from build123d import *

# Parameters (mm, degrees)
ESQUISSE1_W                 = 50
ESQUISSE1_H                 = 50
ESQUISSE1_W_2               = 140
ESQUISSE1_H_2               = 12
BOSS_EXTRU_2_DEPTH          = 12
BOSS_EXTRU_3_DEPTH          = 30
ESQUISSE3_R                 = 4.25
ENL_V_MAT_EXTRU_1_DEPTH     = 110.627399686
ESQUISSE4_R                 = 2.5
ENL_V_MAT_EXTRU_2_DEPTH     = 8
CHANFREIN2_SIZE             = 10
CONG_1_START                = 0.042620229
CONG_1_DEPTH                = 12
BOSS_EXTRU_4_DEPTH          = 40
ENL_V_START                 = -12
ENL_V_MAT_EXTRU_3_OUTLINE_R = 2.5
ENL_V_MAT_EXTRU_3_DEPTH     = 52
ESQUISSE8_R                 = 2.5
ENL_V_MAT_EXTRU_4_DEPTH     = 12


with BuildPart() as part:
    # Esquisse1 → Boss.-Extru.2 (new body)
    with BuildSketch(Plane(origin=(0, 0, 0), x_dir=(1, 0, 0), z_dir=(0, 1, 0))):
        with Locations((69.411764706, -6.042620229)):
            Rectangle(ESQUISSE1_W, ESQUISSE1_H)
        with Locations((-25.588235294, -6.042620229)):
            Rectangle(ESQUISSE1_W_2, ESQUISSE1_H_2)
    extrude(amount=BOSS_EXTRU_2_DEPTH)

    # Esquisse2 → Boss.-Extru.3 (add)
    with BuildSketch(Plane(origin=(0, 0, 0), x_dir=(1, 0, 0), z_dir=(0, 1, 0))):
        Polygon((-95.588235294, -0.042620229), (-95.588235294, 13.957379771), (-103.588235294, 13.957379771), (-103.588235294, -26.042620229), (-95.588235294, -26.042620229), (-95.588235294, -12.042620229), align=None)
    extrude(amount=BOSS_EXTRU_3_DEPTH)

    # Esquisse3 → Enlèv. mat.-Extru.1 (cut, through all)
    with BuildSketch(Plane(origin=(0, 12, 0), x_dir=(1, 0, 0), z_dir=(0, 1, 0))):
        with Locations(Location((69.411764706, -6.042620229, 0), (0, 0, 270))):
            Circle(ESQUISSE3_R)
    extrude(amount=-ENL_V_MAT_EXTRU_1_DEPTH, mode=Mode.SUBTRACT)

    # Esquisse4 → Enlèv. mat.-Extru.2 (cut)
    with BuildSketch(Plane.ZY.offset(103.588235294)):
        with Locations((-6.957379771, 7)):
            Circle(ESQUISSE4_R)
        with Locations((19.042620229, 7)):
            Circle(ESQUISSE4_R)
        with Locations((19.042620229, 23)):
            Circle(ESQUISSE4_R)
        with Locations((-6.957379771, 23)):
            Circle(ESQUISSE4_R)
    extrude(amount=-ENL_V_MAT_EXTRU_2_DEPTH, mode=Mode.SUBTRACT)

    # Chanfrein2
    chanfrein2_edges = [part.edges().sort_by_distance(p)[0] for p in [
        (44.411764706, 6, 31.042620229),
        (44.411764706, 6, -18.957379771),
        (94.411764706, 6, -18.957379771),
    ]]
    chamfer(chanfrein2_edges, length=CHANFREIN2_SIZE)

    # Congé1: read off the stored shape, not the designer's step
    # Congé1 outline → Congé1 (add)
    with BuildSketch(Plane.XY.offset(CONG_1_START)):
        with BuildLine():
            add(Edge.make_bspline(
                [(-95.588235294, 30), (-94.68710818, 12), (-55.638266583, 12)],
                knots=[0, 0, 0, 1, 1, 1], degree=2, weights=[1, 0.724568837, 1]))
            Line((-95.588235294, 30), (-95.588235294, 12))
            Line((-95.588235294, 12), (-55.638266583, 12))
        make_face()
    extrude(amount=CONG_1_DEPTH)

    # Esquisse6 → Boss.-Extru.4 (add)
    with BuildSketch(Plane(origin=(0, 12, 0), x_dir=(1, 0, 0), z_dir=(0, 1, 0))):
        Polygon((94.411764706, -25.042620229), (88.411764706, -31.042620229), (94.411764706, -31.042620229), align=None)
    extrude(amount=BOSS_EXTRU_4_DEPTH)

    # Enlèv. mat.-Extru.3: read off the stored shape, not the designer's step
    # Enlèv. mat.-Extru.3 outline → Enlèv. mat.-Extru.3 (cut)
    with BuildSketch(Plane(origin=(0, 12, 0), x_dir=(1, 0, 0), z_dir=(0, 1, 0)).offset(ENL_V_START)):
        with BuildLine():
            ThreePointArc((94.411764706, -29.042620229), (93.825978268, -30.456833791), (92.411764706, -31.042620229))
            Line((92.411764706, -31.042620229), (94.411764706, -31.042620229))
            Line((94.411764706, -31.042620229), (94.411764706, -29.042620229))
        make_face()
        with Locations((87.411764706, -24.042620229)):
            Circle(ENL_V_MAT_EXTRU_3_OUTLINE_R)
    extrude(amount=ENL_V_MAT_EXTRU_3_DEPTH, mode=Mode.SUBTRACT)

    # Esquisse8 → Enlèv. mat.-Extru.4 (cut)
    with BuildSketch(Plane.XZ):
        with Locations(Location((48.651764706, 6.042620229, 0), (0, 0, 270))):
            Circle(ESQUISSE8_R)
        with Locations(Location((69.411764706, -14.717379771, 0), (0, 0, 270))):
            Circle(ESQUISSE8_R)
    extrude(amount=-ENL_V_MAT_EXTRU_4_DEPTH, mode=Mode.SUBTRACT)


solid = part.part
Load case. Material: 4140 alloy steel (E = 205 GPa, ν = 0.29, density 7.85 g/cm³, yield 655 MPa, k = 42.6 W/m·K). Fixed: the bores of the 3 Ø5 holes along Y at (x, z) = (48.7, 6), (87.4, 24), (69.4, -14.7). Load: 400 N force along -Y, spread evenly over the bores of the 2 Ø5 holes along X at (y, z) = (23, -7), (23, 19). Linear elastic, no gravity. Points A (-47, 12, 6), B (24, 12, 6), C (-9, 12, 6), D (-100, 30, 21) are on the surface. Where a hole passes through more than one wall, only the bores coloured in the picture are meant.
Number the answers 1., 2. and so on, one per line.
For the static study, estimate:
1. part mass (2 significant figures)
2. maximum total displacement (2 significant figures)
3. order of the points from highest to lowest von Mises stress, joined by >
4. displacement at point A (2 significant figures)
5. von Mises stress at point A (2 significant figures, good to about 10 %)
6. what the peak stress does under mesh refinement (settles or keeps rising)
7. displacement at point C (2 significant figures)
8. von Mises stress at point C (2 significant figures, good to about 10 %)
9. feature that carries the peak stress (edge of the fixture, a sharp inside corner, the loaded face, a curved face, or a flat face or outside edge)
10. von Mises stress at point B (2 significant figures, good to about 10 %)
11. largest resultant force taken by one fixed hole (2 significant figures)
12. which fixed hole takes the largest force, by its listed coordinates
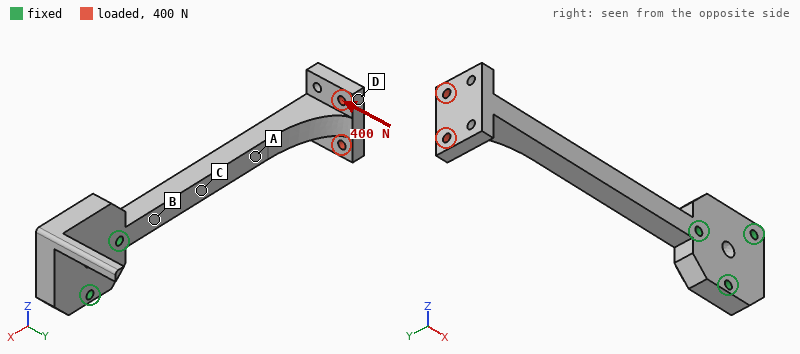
1. 460 g
2. 1.3 mm
3. B > C > A > D
4. 0.58 mm
5. 73 MPa
6. keeps rising
7. 0.23 mm
8. 130 MPa
9. edge of the fixture
10. 170 MPa
11. 840 N
12. (48.7, 6)
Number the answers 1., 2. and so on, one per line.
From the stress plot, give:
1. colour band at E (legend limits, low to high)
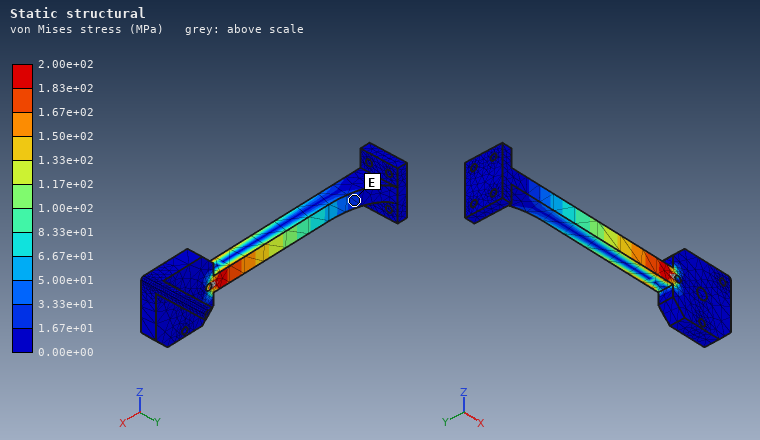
1. 1.67e+01 to 3.33e+01 MPa
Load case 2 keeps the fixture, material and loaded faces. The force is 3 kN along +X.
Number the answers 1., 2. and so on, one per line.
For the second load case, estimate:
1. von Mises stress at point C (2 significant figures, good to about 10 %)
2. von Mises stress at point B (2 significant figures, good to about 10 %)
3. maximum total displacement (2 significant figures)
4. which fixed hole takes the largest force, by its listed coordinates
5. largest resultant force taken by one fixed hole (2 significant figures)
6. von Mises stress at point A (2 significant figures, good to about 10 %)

1. 200 MPa
2. 200 MPa
3. 1.6 mm
4. (48.7, 6)
5. 2.7 kN
6. 200 MPa
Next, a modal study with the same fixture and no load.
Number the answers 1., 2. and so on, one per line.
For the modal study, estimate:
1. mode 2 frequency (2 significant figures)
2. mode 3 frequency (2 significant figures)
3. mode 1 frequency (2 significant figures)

1. 270 Hz
2. 1500 Hz
3. 270 Hz
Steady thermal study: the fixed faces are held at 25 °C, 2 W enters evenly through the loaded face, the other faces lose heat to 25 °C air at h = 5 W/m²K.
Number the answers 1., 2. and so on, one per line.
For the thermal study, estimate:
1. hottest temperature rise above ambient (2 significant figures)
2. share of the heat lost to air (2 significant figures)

1. 29 K
2. 47 %
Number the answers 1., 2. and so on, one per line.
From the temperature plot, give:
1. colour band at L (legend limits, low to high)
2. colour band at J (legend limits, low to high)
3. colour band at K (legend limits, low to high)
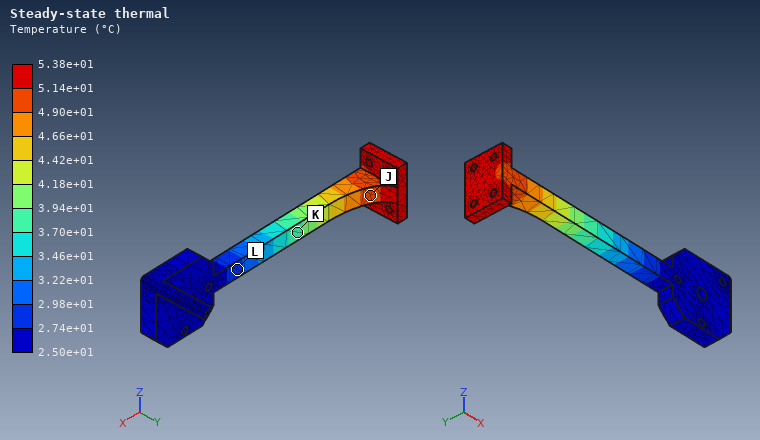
1. 2.74e+01 to 2.98e+01 °C
2. 4.90e+01 to 5.14e+01 °C
3. 3.70e+01 to 3.94e+01 °C
